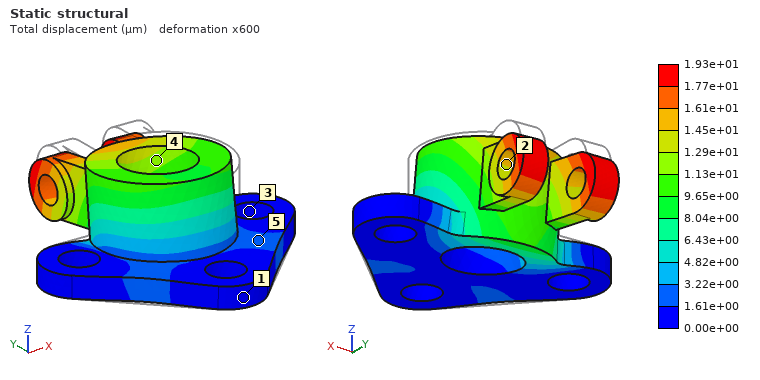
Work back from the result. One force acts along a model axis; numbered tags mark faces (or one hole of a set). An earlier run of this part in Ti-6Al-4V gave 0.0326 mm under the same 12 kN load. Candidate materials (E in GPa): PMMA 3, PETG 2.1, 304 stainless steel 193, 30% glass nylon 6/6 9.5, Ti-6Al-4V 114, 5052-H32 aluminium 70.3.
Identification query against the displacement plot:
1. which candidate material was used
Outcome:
304 stainless steel
